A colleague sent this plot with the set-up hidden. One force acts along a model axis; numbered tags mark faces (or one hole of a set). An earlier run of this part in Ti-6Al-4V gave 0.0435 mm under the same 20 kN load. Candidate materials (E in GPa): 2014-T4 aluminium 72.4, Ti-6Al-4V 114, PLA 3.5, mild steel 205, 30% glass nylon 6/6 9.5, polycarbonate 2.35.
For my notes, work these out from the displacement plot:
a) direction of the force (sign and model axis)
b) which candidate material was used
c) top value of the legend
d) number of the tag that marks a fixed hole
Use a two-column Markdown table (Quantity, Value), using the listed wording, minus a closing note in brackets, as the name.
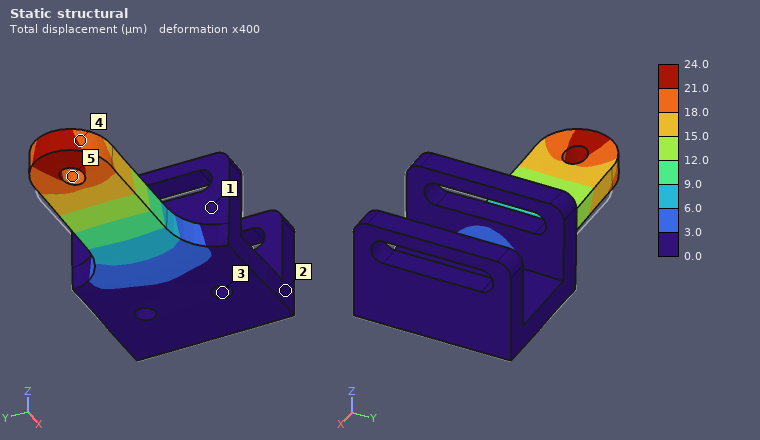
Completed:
| Quantity | Value |
|---|---|
| direction of the force | -X |
| which candidate material was used | mild steel |
| top value of the legend | 24.0 µm |
| number of the tag that marks a fixed hole | 3 |
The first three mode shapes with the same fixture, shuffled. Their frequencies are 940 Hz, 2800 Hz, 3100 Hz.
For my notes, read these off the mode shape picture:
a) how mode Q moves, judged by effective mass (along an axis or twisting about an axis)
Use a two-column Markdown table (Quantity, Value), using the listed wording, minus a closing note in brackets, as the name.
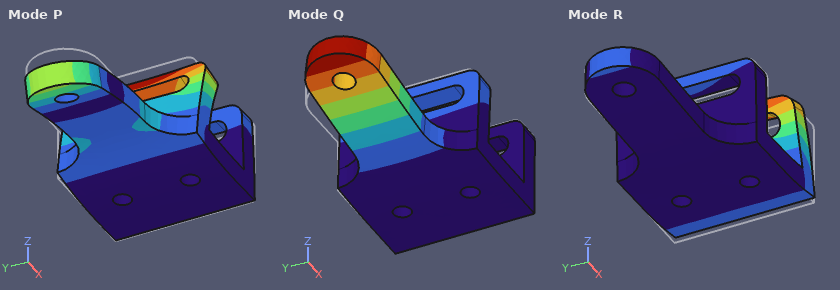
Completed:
| Quantity | Value |
|---|---|
| how mode Q moves, judged by effective mass | along Z |
